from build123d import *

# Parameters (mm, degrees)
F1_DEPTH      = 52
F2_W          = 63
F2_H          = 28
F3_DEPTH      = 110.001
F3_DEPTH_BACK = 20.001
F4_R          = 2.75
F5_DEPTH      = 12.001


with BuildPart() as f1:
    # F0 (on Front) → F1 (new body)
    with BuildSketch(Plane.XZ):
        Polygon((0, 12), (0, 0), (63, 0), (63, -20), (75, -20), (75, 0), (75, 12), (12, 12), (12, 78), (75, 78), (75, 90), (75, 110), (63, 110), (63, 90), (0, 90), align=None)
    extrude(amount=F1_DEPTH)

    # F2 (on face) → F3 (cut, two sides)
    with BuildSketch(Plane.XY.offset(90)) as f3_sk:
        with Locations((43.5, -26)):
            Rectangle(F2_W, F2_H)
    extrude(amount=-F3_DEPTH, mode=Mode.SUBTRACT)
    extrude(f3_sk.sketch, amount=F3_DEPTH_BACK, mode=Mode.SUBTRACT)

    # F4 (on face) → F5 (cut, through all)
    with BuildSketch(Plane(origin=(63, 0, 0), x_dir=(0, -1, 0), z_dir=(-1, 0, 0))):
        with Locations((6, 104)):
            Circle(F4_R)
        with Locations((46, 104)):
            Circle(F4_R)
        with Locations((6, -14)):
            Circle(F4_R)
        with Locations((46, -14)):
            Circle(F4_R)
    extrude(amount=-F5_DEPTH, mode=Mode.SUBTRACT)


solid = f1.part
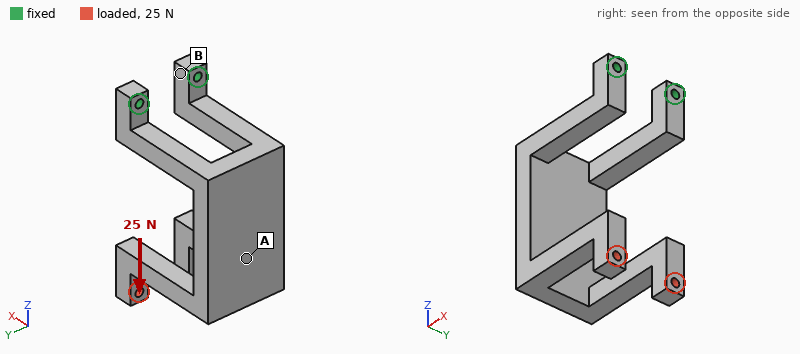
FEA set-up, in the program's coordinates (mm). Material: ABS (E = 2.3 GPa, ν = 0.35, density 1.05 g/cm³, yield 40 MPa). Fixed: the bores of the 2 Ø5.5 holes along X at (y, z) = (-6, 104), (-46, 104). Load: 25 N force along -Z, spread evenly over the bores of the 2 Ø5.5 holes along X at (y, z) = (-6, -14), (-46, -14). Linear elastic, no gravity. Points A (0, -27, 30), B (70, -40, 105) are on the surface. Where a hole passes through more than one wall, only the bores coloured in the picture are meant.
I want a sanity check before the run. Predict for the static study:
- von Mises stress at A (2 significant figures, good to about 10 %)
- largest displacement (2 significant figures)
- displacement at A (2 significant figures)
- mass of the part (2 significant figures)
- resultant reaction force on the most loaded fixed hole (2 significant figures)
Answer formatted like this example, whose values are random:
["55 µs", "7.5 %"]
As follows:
["1.2 MPa", "1.6 mm", "0.49 mm", "110 g", "13 N"]
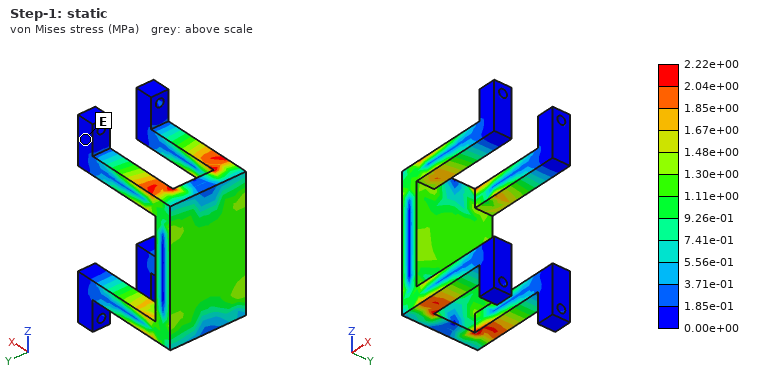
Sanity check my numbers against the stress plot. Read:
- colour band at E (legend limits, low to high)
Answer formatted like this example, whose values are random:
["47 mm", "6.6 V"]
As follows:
["0.00e+00 to 1.85e-01 MPa"]
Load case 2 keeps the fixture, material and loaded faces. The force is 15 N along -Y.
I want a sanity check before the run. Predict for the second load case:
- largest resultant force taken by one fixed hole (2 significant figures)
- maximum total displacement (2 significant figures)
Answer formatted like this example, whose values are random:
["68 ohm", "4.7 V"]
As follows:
["20 N", "1.8 mm"]
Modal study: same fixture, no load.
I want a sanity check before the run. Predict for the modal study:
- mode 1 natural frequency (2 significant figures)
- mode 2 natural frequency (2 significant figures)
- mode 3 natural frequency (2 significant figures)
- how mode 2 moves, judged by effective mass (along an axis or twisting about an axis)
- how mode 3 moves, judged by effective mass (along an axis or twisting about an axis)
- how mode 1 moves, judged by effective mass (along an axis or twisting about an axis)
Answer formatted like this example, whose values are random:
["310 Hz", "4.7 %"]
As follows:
["76 Hz", "99 Hz", "210 Hz", "along Y", "along Z", "along X"]
